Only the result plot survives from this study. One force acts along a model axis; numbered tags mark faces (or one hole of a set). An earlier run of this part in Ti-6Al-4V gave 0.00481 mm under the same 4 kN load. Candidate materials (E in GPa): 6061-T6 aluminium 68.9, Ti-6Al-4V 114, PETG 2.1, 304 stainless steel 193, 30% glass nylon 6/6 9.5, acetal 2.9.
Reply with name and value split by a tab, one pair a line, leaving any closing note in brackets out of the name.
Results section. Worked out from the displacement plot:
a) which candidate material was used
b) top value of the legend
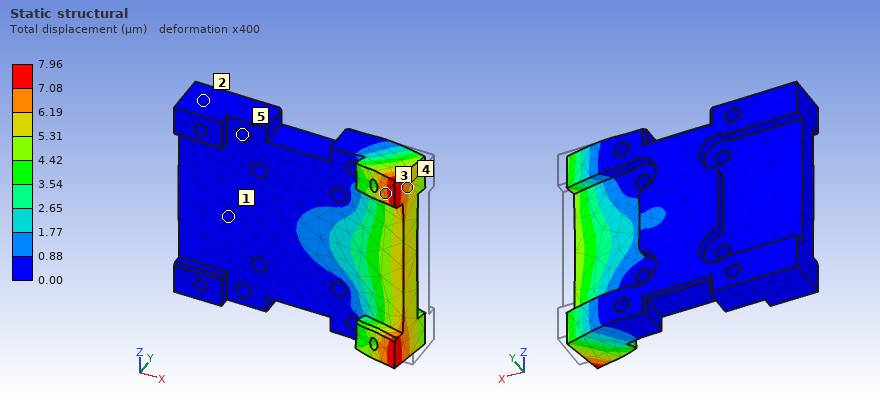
which candidate material was used	6061-T6 aluminium
top value of the legend	7.96 µm
